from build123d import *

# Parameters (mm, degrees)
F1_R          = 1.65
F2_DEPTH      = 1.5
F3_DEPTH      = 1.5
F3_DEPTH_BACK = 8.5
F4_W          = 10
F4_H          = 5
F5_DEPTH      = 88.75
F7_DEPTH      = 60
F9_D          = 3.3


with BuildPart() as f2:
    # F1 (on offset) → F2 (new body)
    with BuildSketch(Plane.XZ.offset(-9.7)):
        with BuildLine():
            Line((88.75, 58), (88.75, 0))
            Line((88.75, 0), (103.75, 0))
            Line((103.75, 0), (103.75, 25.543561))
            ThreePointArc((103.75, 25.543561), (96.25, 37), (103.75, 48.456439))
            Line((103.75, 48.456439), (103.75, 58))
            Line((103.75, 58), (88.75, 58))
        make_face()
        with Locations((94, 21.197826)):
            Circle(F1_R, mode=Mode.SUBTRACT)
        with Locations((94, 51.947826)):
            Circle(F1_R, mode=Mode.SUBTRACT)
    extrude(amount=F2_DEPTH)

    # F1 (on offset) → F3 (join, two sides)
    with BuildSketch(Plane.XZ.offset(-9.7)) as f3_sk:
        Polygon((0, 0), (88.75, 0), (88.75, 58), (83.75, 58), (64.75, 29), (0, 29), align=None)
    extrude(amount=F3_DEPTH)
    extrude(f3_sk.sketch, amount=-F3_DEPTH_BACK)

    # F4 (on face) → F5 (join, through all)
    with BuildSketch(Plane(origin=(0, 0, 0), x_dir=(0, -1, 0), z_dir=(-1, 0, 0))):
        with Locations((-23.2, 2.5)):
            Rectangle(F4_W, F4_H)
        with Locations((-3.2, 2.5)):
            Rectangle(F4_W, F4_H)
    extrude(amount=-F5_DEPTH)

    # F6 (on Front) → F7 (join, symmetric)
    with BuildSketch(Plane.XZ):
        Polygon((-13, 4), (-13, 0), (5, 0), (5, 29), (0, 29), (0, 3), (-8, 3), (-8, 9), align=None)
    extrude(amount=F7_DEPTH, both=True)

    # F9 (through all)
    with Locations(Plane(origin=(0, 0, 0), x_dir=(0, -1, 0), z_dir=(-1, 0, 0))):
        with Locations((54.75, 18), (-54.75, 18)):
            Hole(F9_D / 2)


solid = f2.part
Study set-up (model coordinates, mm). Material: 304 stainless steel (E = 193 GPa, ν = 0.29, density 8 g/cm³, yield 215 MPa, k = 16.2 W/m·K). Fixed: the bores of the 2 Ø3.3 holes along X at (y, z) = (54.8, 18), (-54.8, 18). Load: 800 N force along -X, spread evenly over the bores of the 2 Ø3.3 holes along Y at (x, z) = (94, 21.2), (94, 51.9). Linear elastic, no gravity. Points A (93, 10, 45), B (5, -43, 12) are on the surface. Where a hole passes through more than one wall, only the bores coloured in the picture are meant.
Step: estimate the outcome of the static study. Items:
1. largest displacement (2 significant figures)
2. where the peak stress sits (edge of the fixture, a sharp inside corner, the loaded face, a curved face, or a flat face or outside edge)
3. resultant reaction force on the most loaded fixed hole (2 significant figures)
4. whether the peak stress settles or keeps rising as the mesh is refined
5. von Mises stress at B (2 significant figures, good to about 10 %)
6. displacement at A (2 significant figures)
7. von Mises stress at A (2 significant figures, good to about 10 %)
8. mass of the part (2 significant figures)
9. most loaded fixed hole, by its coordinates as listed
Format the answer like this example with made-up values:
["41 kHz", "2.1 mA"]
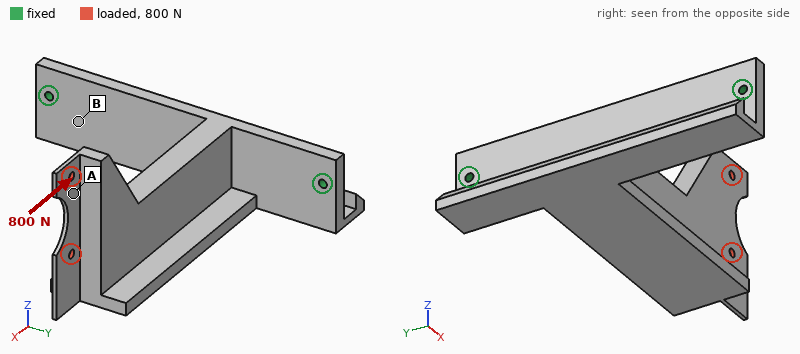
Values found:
["0.57 mm", "edge of the fixture", "500 N", "keeps rising", "47 MPa", "0.49 mm", "12 MPa", "500 g", "(54.8, 18)"]
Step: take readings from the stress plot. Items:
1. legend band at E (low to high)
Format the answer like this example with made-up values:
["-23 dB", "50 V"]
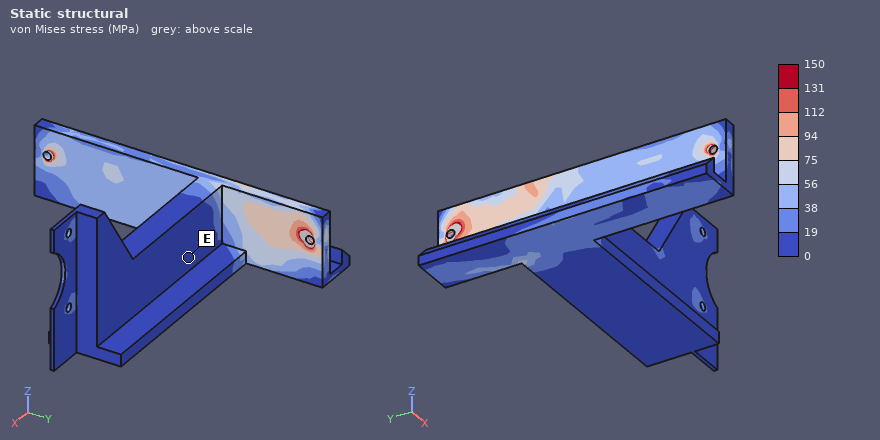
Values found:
["0 to 19 MPa"]
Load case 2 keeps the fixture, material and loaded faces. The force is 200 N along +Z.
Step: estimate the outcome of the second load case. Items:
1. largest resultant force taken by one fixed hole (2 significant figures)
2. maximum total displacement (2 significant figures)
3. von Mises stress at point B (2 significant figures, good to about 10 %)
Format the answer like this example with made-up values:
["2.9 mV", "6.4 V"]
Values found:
["250 N", "0.46 mm", "40 MPa"]
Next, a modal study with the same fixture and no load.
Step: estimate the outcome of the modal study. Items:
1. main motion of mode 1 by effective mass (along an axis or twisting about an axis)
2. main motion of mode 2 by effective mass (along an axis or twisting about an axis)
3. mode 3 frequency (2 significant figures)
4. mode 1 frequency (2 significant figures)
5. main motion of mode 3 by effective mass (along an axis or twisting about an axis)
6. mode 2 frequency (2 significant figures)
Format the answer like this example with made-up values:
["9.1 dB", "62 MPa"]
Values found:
["along Z", "along Y", "1400 Hz", "330 Hz", "along X", "880 Hz"]
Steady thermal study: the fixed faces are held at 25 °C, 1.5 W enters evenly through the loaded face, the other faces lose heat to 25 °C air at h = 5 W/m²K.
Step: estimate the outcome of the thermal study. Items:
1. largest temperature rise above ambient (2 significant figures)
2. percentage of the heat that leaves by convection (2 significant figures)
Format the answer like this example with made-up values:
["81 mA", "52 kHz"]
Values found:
["38 K", "67 %"]
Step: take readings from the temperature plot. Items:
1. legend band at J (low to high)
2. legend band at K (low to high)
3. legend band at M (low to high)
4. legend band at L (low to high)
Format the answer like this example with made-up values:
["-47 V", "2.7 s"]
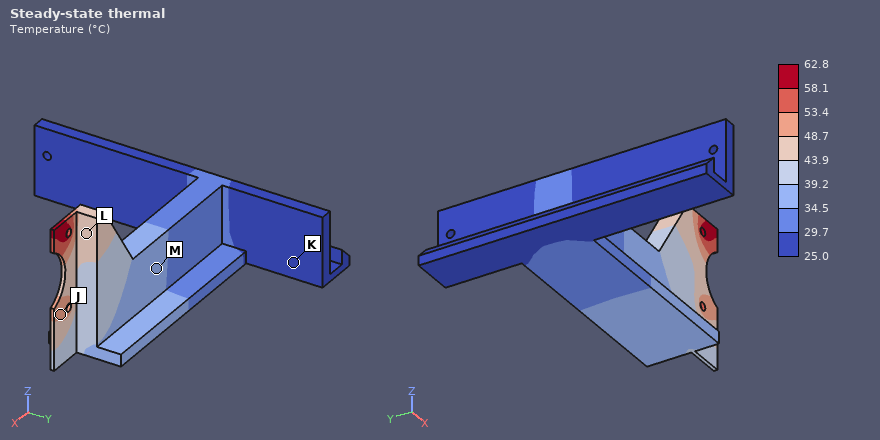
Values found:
["48.7 to 53.4 °C", "25.0 to 29.7 °C", "34.5 to 39.2 °C", "43.9 to 48.7 °C"]
